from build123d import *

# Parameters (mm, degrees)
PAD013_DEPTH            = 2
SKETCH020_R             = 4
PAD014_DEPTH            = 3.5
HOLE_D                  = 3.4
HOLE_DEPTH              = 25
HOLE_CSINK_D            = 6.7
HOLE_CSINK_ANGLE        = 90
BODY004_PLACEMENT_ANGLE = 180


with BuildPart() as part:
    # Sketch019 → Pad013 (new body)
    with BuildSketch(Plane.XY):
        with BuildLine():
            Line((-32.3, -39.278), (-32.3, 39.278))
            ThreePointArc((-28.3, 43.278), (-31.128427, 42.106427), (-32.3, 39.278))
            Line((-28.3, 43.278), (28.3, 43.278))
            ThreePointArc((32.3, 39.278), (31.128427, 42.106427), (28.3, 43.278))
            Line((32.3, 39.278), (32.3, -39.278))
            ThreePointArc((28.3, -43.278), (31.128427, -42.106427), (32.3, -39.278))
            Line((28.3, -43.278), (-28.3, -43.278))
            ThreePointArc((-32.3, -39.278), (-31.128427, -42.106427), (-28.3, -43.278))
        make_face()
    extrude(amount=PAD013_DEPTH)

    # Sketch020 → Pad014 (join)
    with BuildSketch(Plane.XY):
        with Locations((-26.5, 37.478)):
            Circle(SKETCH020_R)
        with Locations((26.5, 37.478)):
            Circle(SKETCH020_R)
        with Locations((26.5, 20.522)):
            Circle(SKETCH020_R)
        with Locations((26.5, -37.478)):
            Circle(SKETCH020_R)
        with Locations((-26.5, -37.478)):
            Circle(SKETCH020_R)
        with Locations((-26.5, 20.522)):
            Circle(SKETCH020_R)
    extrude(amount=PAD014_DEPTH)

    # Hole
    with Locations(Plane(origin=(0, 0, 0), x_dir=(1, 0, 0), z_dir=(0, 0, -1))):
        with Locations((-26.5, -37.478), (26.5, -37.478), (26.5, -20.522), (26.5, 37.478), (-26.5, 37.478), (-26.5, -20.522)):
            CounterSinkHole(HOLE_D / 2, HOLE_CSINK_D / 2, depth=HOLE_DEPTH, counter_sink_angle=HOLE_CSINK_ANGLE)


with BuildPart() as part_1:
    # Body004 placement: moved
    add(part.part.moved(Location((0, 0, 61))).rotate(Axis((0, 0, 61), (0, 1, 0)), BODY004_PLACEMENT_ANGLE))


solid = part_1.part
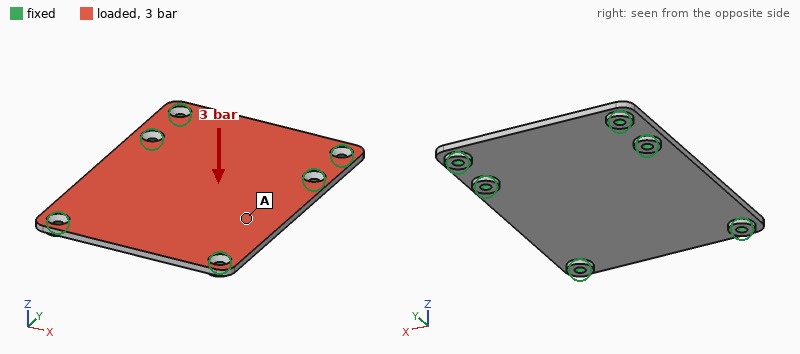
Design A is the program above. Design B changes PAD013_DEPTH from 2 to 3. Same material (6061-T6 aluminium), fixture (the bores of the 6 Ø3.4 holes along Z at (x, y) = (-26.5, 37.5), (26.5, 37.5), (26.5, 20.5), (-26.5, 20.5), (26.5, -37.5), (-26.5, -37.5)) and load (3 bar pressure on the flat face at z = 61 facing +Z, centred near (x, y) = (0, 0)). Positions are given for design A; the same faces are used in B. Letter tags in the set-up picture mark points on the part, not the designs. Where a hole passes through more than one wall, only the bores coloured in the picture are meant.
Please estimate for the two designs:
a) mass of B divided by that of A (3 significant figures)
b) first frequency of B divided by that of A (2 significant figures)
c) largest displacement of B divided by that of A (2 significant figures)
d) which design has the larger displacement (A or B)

1.47
1.3
0.38
A
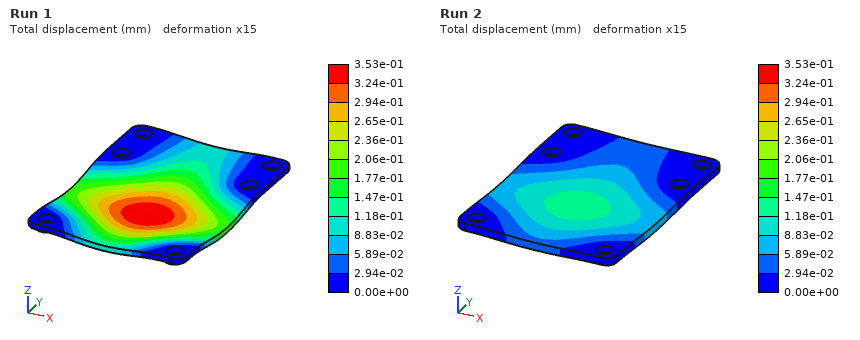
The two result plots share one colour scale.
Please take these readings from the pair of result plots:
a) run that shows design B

Run 2
